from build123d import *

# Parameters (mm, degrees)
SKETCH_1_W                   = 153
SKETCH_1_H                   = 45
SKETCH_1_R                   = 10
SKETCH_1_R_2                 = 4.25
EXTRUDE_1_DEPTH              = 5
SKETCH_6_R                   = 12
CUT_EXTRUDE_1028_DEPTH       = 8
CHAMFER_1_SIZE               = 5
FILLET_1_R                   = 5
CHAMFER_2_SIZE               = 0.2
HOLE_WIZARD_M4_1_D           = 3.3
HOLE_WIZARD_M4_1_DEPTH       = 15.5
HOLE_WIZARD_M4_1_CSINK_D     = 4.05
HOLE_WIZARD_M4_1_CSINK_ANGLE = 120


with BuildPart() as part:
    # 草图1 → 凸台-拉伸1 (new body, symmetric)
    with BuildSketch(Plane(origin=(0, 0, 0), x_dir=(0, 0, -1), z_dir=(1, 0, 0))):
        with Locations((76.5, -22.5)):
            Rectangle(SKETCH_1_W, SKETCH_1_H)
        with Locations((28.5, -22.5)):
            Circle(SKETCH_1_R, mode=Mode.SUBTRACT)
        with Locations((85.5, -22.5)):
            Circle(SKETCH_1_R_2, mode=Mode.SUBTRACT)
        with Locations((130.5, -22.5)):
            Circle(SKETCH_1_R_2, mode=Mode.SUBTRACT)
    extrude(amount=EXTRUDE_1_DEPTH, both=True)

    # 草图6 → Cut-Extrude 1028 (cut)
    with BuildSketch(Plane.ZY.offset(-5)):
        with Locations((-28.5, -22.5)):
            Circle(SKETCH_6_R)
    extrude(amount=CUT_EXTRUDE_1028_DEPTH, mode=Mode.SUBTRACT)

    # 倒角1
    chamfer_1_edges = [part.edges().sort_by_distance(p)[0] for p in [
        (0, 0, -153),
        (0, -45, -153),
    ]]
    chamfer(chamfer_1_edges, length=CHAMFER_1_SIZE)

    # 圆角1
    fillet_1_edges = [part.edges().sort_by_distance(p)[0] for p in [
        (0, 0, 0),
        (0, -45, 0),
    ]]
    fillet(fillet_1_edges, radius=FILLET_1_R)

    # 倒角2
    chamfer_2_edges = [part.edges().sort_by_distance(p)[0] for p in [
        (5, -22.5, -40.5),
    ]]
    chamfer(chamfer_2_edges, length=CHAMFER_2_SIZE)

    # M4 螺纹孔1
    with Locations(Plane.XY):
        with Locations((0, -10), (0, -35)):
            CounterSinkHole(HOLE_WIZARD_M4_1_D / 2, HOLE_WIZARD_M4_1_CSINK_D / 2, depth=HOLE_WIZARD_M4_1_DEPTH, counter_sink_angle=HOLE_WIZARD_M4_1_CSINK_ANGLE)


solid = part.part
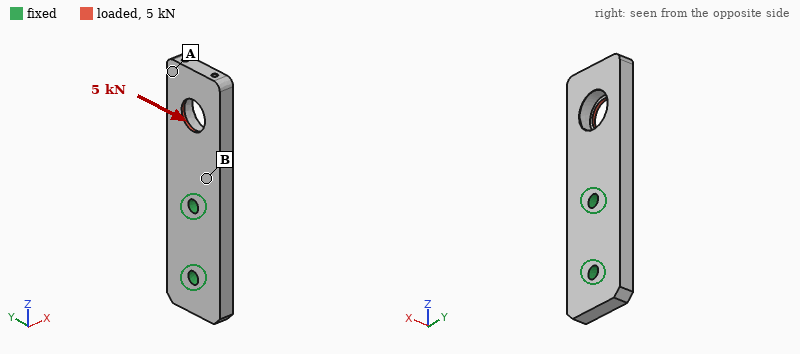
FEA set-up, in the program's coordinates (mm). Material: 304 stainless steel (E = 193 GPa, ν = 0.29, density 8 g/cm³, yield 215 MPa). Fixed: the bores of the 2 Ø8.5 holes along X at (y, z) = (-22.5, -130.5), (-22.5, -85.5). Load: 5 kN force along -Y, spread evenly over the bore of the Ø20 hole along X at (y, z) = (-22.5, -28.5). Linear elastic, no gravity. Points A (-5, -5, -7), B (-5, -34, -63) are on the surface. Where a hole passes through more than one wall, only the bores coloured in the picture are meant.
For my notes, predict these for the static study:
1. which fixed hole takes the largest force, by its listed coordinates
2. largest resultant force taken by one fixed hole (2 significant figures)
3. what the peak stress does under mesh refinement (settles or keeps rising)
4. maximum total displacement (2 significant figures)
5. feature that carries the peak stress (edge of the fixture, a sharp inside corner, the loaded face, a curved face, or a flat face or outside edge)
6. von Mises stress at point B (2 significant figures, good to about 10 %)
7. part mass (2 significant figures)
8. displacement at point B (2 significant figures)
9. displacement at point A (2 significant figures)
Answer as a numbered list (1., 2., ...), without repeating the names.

1. (-22.5, -85.5)
2. 9.6 kN
3. keeps rising
4. 0.10 mm
5. edge of the fixture
6. 50 MPa
7. 500 g
8. 0.021 mm
9. 0.094 mm
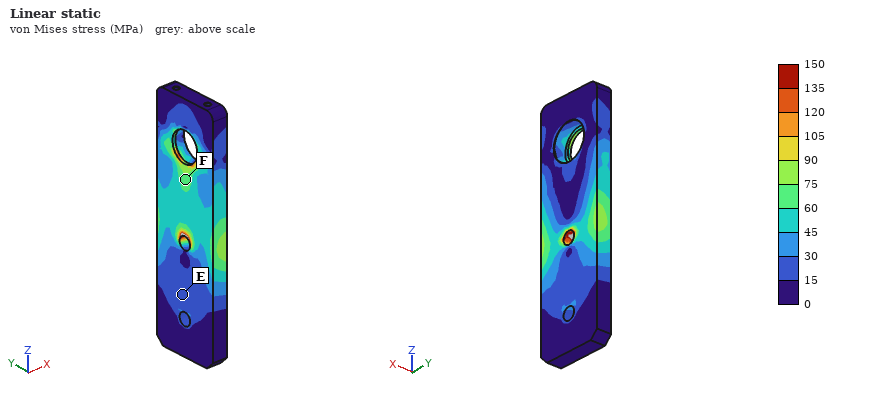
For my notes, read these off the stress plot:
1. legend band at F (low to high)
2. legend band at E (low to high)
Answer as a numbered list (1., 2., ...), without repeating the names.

1. 60 to 75 MPa
2. 15 to 30 MPa
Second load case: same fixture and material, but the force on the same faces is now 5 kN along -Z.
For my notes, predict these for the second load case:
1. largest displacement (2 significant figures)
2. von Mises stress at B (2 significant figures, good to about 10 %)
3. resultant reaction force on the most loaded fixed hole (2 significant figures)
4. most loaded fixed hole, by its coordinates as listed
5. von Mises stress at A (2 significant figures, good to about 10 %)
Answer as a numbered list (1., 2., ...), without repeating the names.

1. 98 µm
2. 37 MPa
3. 4.2 kN
4. (-22.5, -85.5)
5. 6.7 MPa
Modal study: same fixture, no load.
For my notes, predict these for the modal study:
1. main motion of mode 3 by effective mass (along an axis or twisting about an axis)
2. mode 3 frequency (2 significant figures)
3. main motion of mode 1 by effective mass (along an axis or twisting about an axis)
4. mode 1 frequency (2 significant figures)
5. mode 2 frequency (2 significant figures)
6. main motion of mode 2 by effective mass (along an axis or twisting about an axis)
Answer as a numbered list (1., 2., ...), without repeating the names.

1. twisting about Z
2. 3500 Hz
3. along X
4. 1100 Hz
5. 3300 Hz
6. along Y
